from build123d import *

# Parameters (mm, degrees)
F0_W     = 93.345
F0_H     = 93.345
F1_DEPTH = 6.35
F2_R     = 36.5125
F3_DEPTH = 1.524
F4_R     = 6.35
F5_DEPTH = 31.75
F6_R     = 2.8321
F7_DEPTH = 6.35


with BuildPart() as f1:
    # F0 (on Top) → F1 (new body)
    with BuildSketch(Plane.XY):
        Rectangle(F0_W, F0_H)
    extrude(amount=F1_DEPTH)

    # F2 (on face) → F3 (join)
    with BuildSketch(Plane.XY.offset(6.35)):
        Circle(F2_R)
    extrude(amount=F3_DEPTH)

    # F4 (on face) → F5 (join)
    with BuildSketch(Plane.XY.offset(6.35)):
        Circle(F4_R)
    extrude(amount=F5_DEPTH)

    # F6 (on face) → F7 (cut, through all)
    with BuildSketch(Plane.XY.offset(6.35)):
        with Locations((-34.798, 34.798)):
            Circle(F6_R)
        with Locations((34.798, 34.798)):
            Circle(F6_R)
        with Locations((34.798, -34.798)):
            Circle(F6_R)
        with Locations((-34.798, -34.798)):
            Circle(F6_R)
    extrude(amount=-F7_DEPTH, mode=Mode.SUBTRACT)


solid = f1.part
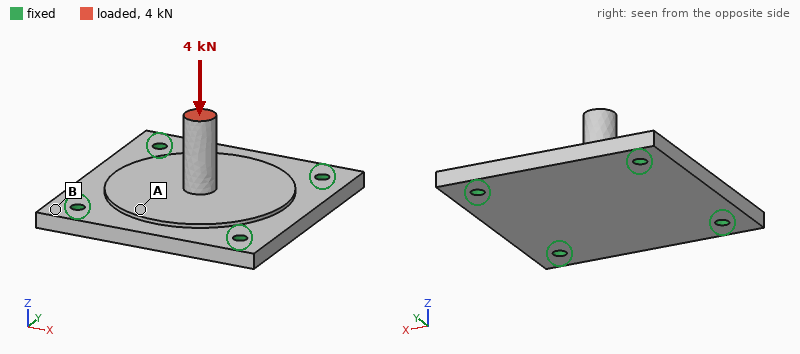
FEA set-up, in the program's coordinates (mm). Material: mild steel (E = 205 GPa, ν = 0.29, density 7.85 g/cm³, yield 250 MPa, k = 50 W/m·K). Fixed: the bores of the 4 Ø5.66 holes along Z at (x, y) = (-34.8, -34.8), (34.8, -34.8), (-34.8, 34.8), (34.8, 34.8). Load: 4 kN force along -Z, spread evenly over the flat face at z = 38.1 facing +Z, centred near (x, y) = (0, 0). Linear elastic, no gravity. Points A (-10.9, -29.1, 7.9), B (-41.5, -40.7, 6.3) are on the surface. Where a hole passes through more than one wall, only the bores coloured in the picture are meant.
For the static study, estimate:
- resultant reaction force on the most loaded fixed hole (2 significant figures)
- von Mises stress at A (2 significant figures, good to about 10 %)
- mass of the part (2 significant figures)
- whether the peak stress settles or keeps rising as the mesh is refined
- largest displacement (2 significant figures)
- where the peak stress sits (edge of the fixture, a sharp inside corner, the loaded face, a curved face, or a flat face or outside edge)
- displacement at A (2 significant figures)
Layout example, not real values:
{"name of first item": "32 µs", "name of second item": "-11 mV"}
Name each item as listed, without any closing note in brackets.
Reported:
{"resultant reaction force on the most loaded fixed hole": "1.2 kN", "von Mises stress at A": "26 MPa", "mass of the part": "510 g", "whether the peak stress settles or keeps rising as the mesh is refined": "keeps rising", "largest displacement": "39 µm", "where the peak stress sits": "edge of the fixture", "displacement at A": "15 µm"}
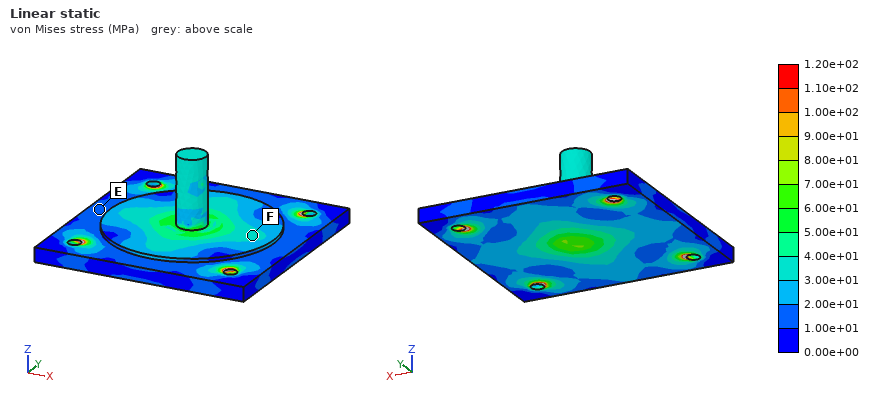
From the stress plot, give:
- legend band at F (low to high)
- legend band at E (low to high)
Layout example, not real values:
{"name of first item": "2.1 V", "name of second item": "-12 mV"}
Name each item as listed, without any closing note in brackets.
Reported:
{"legend band at F": "3.00e+01 to 4.00e+01 MPa", "legend band at E": "1.00e+01 to 2.00e+01 MPa"}
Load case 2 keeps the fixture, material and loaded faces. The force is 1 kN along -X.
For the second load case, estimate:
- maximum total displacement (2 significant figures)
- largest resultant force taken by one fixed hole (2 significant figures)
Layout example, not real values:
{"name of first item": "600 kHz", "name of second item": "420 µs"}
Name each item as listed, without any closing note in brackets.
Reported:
{"maximum total displacement": "67 µm", "largest resultant force taken by one fixed hole": "420 N"}
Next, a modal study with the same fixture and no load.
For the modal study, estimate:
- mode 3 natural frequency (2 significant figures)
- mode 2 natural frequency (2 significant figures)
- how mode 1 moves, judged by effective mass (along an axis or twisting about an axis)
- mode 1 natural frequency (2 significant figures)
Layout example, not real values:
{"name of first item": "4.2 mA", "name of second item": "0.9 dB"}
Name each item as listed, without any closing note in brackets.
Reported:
{"mode 3 natural frequency": "6000 Hz", "mode 2 natural frequency": "6000 Hz", "how mode 1 moves, judged by effective mass": "along Z", "mode 1 natural frequency": "4400 Hz"}
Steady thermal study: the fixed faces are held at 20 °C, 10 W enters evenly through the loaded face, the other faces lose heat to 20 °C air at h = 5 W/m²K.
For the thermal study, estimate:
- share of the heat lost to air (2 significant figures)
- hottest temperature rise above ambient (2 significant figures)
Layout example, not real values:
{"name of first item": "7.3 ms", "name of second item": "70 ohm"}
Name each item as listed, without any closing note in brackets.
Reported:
{"share of the heat lost to air": "5.9 %", "hottest temperature rise above ambient": "61 K"}
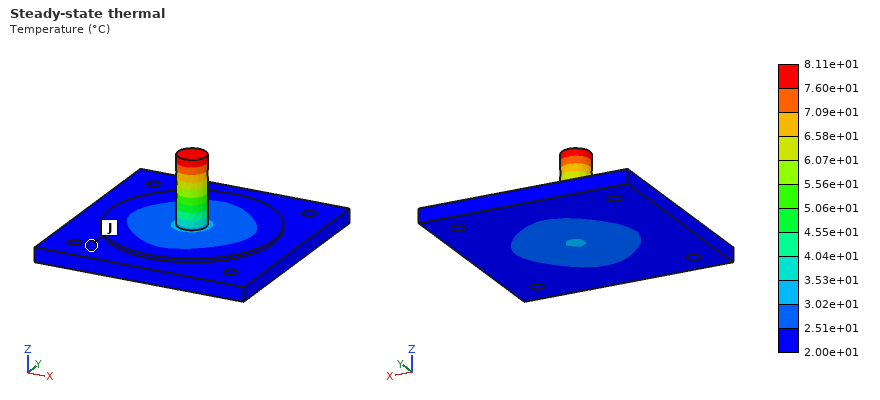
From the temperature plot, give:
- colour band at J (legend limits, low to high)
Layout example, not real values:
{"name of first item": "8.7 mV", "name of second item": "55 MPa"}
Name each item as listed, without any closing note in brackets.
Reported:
{"colour band at J": "2.00e+01 to 2.51e+01 °C"}
